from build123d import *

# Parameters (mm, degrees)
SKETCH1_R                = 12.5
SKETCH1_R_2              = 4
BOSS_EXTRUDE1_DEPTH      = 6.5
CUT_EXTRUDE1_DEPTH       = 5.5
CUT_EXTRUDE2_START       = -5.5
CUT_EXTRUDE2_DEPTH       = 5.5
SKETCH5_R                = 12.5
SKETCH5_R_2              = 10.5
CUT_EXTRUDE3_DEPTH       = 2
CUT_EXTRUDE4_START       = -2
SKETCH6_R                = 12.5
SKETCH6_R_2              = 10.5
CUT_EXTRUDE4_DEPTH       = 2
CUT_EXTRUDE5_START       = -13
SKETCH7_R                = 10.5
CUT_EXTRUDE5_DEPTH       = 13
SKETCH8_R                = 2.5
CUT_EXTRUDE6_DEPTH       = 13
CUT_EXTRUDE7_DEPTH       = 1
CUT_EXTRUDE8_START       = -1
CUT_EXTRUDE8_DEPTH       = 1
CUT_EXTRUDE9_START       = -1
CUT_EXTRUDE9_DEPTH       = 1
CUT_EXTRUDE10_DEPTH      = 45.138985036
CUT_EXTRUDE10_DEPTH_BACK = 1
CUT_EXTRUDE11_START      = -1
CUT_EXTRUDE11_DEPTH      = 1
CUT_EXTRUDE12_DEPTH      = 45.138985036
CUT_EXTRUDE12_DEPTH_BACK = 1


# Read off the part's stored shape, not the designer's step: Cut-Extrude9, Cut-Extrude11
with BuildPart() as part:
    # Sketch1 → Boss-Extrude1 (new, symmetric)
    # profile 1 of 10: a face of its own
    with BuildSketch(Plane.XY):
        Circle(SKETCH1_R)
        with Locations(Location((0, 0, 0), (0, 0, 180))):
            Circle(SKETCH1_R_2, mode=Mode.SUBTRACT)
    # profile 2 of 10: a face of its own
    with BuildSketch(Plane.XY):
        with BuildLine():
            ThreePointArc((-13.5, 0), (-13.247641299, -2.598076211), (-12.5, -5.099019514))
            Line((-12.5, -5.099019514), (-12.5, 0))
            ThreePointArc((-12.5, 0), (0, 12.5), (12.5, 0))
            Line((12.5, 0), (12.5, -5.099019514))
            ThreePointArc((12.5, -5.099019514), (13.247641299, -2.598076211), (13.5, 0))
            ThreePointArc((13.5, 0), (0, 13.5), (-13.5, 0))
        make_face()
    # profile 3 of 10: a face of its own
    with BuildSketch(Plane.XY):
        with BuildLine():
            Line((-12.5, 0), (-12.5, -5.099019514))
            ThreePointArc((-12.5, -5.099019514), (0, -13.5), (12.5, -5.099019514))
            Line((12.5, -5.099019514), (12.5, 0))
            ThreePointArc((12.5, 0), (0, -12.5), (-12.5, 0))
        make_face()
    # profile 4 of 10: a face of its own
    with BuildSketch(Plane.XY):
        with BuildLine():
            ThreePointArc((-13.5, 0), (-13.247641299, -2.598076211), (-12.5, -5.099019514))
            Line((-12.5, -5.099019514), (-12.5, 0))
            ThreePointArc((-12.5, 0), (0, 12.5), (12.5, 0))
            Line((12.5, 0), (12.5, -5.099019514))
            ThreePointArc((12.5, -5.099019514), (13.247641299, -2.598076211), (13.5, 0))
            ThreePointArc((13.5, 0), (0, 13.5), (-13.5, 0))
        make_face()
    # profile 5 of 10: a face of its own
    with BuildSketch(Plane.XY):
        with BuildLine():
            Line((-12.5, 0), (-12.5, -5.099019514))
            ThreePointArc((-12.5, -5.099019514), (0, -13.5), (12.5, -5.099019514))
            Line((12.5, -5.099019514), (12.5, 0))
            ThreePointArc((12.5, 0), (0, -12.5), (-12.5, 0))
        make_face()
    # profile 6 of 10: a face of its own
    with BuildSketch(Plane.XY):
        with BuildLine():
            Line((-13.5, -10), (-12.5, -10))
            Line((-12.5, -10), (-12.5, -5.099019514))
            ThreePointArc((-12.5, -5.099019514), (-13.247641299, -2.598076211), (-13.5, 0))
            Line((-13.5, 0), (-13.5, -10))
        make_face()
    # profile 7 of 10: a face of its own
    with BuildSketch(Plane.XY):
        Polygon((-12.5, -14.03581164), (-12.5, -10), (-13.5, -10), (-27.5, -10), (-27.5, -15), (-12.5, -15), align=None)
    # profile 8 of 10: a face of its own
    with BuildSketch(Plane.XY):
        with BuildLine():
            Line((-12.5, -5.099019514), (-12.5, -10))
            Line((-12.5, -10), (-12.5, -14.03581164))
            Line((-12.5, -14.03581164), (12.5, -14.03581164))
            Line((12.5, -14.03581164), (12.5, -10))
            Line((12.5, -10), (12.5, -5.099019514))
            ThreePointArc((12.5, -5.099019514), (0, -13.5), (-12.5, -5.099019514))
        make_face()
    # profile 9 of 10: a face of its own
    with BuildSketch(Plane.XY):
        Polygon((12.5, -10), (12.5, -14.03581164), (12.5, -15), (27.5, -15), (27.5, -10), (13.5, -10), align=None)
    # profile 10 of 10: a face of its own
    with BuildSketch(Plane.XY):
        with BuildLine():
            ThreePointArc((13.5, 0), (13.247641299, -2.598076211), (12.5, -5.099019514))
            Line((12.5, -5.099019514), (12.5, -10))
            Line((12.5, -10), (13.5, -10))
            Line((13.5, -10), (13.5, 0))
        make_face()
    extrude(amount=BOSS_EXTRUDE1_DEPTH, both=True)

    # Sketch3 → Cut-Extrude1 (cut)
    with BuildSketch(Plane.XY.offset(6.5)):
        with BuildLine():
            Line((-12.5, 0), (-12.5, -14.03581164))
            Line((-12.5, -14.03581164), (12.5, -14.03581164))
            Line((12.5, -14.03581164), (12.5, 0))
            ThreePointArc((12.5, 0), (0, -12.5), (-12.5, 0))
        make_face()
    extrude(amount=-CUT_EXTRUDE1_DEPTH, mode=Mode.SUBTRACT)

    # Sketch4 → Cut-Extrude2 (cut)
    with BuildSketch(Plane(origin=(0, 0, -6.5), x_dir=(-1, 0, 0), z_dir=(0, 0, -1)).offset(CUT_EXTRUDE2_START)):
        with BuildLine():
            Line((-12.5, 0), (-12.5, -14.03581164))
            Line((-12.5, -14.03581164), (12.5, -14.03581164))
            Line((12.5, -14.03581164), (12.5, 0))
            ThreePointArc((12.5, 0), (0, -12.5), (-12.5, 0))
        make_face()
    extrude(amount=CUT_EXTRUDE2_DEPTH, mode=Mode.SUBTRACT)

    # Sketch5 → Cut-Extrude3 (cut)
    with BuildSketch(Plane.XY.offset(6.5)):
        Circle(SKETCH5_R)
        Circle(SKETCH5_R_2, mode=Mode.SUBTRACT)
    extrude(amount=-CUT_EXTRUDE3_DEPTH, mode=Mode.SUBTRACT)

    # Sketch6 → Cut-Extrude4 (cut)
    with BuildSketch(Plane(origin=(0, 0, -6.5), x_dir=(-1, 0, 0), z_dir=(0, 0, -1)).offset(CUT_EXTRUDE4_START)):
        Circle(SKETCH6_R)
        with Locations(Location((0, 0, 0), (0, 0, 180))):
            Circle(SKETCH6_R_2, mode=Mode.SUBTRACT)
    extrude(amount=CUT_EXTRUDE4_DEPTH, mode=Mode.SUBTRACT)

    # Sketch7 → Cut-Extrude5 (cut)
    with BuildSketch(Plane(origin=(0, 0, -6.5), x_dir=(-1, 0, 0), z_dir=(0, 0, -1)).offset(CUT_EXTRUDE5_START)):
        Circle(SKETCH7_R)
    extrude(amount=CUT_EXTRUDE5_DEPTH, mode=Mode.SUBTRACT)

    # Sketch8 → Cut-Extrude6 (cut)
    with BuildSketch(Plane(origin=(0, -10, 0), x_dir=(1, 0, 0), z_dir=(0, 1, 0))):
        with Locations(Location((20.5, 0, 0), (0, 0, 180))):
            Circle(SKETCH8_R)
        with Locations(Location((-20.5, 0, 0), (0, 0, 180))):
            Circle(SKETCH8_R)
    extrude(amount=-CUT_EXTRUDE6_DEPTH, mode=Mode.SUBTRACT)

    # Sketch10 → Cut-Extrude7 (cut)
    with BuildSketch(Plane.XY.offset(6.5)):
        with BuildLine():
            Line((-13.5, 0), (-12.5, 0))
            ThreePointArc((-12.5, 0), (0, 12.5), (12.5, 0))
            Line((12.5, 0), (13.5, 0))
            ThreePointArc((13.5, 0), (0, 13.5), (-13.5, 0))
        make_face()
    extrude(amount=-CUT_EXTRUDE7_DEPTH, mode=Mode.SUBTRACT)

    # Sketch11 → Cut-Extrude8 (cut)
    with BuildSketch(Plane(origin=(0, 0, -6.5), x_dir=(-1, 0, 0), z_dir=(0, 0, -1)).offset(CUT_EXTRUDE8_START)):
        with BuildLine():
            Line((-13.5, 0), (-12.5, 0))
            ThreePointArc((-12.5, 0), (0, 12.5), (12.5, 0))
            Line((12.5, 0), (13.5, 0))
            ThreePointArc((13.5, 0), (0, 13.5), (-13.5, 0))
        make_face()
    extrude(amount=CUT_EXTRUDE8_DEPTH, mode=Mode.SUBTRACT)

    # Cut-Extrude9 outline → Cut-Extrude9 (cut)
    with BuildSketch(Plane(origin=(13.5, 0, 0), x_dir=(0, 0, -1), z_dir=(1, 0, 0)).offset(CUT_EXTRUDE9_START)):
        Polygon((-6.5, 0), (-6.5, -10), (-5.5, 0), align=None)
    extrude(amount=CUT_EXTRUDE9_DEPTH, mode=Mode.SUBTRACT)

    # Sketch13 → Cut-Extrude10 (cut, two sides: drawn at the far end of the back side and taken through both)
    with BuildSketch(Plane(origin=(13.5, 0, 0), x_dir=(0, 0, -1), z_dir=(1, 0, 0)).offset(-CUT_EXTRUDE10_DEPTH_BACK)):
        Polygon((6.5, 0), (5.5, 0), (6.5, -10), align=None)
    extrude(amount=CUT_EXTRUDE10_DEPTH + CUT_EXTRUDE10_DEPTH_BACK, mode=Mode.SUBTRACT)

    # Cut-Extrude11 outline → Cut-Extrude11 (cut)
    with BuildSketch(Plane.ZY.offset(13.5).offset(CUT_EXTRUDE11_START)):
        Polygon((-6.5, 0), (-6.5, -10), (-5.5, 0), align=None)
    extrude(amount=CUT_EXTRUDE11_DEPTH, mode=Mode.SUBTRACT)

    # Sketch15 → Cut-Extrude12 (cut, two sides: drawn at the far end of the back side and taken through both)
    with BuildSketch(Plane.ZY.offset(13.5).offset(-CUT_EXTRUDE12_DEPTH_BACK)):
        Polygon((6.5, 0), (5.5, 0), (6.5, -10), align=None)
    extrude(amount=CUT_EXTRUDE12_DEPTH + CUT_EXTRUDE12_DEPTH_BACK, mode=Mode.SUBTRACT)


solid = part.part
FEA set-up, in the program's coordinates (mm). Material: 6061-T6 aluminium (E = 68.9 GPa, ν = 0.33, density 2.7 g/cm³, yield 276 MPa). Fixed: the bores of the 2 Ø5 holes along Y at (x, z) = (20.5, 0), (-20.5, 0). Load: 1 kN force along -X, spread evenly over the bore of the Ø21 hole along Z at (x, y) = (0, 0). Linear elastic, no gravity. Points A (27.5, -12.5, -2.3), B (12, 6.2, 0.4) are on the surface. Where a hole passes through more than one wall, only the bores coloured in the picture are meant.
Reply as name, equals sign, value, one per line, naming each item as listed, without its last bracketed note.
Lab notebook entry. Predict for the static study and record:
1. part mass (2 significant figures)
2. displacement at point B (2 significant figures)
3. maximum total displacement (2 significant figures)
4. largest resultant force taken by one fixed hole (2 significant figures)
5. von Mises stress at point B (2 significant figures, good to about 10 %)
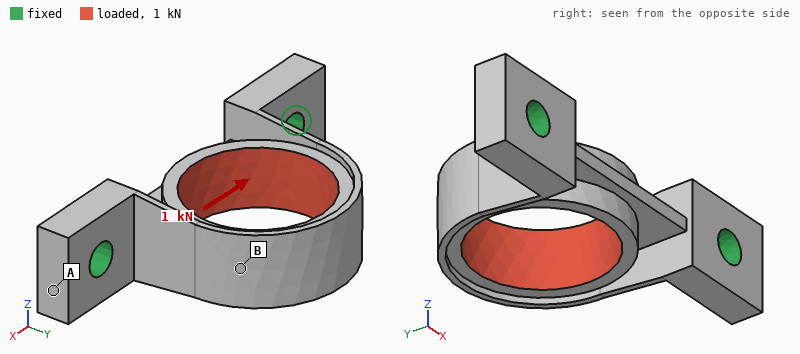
part mass = 11 g
displacement at point B = 81 µm
maximum total displacement = 91 µm
largest resultant force taken by one fixed hole = 630 N
von Mises stress at point B = 45 MPa
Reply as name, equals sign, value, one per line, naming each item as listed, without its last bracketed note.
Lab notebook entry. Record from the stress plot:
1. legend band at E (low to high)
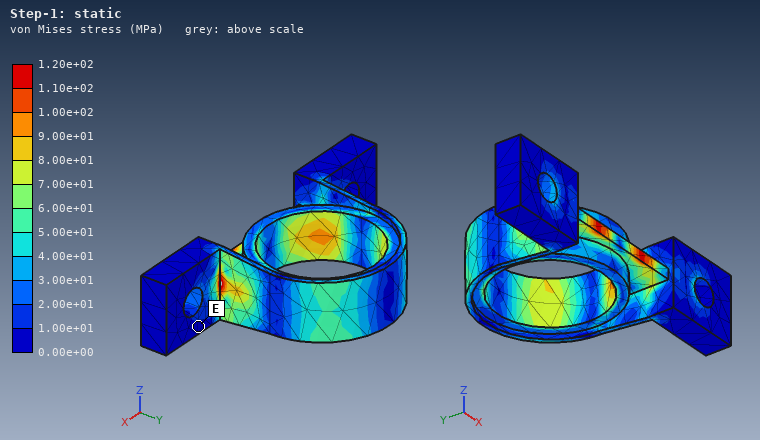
legend band at E = 0.00e+00 to 1.00e+01 MPa
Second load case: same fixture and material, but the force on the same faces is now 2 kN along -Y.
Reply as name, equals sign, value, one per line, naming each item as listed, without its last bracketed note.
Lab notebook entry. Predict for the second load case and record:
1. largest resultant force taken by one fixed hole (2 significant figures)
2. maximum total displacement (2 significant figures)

largest resultant force taken by one fixed hole = 1.0 kN
maximum total displacement = 41 µm
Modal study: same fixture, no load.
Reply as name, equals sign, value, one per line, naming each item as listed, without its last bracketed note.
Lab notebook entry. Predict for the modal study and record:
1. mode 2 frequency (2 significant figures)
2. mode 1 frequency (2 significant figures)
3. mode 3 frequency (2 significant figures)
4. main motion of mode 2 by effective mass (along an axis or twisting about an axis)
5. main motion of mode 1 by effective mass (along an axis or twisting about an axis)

mode 2 frequency = 7500 Hz
mode 1 frequency = 5400 Hz
mode 3 frequency = 12 kHz
main motion of mode 2 by effective mass = along X
main motion of mode 1 by effective mass = along Z
